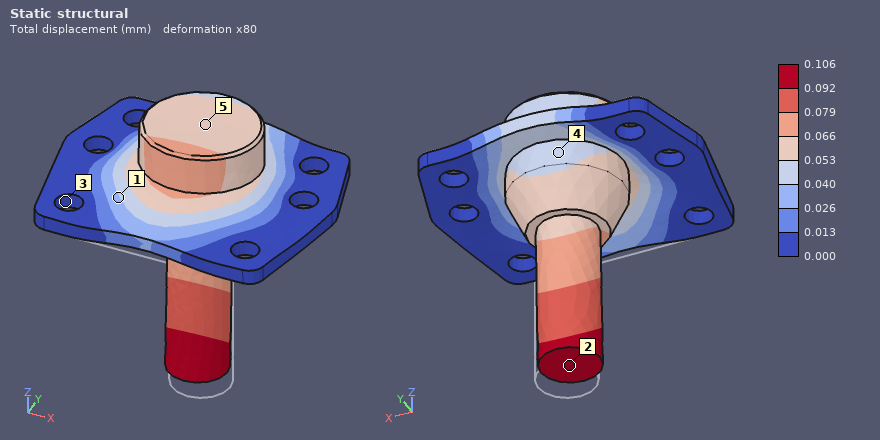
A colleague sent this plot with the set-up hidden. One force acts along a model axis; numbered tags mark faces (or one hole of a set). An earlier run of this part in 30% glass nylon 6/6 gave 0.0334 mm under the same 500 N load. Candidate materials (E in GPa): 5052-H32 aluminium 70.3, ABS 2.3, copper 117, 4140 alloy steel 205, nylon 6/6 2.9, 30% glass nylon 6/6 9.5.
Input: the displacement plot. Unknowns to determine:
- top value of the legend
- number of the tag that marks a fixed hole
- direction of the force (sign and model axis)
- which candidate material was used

0.106 mm
3
+Z
nylon 6/6
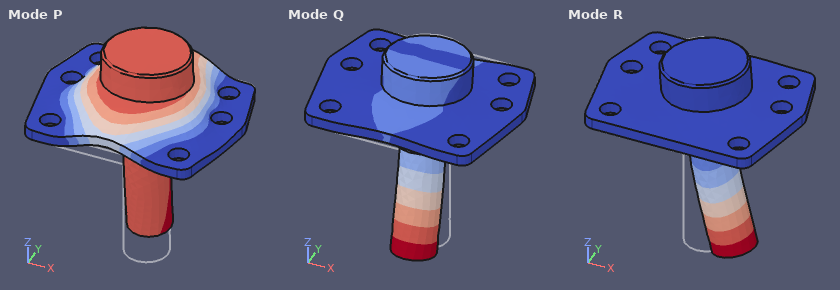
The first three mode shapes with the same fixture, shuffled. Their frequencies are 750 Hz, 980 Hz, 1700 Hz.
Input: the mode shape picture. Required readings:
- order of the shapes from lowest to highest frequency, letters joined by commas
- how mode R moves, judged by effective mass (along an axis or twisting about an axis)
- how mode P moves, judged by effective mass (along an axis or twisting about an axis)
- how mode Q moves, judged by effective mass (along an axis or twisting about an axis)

Q, R, P
along X
along Z
along Y
